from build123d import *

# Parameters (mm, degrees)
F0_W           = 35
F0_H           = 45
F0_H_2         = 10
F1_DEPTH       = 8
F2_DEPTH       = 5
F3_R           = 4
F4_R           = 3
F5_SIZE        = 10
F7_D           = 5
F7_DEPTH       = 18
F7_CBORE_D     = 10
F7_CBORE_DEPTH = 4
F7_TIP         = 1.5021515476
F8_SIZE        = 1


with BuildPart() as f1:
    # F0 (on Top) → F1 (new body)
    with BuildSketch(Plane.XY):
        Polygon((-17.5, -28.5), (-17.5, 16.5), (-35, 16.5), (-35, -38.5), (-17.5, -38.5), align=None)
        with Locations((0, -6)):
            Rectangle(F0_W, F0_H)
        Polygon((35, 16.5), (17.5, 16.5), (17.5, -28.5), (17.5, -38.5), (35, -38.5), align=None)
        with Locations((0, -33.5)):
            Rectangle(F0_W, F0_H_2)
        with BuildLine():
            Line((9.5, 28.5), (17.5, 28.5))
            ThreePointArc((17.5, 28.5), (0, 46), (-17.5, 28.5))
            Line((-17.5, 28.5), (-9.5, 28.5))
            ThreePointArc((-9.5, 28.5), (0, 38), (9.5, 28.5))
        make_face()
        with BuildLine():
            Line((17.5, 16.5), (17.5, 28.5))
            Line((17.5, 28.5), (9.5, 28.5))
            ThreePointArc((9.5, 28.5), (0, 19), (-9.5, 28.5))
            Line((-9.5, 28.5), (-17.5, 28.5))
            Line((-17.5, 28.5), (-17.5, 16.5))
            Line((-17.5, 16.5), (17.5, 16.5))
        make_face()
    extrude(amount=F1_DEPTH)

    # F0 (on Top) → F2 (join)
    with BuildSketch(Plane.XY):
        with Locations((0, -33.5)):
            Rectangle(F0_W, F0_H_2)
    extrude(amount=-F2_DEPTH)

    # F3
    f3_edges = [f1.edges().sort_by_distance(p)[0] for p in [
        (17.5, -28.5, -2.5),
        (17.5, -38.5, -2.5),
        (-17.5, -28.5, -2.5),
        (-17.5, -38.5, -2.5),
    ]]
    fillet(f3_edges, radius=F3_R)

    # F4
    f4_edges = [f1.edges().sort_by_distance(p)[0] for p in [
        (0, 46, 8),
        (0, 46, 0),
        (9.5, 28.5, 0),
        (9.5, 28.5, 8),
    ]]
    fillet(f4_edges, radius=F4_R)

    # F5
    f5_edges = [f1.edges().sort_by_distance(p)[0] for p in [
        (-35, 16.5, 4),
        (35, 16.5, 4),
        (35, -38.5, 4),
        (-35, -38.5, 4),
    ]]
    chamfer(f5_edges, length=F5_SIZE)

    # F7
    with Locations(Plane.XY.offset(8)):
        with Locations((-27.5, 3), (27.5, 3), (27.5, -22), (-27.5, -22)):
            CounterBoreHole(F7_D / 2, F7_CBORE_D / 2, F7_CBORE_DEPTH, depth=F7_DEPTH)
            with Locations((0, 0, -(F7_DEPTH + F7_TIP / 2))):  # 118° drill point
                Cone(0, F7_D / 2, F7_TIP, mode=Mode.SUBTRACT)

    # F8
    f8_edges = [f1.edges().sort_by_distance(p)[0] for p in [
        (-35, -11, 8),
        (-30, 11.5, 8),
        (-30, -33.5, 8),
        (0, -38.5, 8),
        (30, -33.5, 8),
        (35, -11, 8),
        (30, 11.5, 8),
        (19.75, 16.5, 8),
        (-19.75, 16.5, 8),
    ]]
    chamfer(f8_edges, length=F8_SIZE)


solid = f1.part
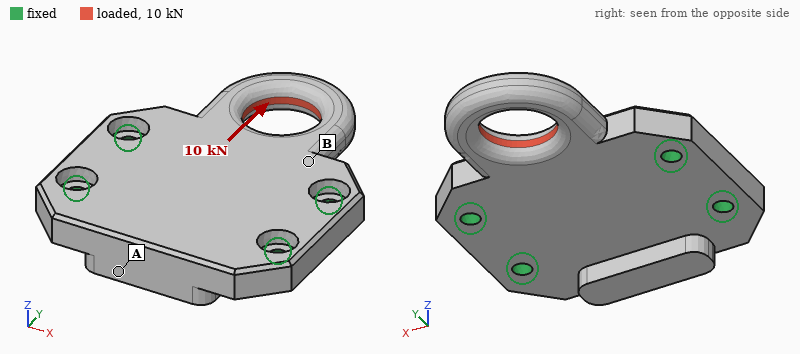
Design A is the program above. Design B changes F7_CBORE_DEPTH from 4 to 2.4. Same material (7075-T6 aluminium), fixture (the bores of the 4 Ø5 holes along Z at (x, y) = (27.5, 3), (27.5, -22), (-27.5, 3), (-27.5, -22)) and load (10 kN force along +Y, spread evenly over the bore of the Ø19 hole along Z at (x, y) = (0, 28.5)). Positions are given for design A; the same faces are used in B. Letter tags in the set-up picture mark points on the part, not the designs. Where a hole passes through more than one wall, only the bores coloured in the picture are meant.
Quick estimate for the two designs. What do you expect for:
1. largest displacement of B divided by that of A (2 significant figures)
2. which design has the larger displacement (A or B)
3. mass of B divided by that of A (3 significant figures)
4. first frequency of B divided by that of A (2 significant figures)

0.88
A
1.01
1.0
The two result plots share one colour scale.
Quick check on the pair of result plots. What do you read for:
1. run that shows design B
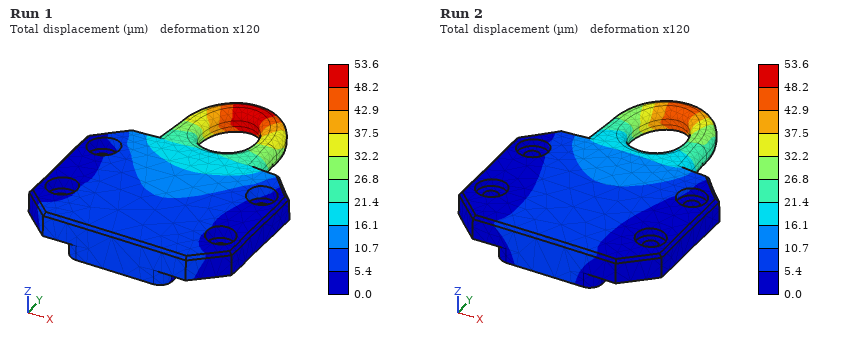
Run 2
